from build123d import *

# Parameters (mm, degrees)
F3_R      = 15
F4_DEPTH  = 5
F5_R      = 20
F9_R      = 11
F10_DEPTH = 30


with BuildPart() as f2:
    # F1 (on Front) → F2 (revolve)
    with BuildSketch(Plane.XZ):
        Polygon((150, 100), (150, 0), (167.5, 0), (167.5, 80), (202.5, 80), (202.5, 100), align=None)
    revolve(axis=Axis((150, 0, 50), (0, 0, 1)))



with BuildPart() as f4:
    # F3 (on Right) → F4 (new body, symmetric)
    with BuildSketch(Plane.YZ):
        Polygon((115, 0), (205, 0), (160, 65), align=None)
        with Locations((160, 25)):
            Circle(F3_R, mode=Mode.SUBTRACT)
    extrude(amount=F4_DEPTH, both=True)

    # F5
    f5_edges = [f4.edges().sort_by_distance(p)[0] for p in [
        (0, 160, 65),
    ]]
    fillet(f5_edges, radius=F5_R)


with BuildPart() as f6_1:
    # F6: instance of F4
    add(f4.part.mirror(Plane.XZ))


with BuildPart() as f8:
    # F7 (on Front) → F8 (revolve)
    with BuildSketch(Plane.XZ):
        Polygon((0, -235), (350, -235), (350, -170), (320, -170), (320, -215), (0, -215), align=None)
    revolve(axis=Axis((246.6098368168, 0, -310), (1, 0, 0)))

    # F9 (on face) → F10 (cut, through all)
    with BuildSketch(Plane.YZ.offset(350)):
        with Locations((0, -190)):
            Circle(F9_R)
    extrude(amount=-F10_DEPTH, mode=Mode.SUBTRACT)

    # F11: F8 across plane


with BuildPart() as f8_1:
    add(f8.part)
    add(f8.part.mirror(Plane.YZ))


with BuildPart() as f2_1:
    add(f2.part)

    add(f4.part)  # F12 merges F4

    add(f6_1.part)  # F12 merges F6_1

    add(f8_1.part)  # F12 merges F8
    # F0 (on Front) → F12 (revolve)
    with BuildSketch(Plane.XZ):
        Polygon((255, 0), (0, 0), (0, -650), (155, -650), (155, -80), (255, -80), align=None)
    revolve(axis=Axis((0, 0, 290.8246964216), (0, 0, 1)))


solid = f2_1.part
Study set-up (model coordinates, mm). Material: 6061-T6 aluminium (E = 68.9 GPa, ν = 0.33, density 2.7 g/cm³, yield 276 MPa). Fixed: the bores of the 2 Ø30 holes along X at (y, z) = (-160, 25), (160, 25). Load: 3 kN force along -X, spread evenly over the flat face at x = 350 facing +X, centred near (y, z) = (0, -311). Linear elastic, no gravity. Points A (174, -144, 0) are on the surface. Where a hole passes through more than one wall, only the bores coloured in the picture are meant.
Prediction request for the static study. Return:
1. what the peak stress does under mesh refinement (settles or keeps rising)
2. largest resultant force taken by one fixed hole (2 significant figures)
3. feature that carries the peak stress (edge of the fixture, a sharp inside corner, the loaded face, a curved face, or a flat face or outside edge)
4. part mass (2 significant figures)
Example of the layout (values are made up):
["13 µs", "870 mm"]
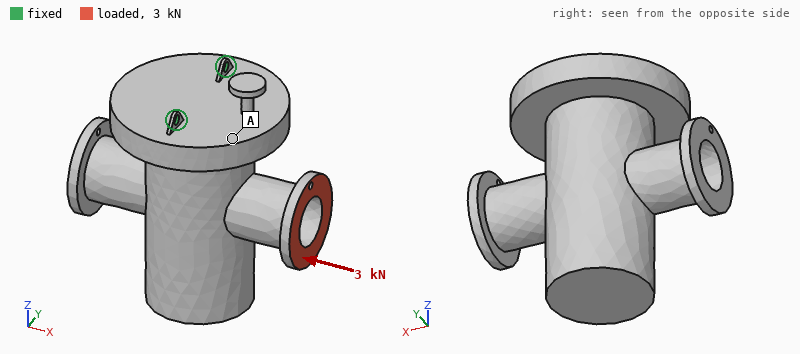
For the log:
["keeps rising", "1.5 kN", "edge of the fixture", "180 kg"]
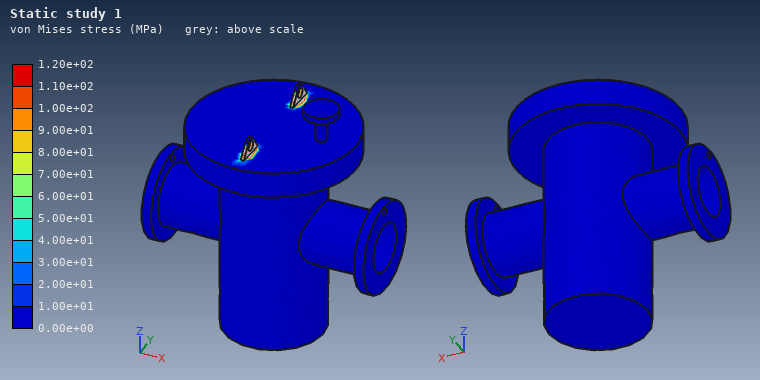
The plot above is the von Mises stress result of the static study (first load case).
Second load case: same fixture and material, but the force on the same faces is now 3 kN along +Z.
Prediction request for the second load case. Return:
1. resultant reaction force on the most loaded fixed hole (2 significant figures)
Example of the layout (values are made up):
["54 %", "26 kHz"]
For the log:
["1.5 kN"]
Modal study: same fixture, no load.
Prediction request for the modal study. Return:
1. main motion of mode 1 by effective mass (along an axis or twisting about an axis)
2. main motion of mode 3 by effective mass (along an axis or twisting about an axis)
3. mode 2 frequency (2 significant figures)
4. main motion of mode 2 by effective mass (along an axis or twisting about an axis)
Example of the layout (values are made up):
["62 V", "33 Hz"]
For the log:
["along X", "twisting about Z", "230 Hz", "along Y"]
